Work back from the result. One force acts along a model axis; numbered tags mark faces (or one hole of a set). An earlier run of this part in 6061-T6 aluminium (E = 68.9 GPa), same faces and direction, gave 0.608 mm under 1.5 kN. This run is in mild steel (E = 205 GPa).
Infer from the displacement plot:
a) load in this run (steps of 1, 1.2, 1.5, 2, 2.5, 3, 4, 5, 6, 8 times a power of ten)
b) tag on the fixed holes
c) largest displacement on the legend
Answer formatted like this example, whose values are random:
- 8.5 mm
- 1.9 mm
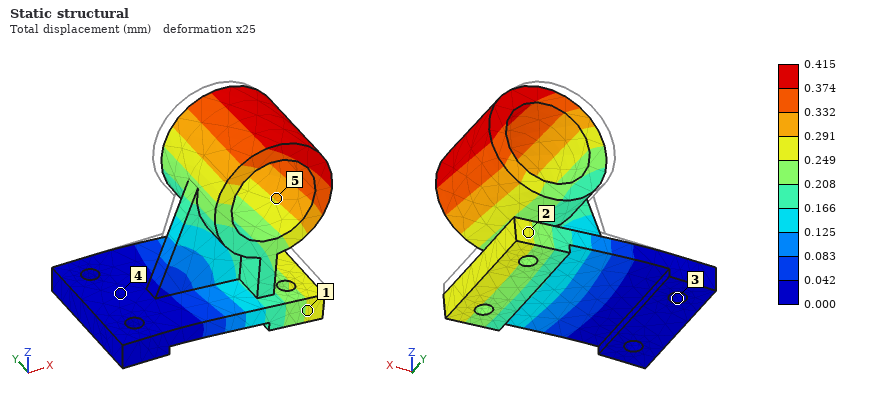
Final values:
- 3 kN
- 3
- 0.415 mm
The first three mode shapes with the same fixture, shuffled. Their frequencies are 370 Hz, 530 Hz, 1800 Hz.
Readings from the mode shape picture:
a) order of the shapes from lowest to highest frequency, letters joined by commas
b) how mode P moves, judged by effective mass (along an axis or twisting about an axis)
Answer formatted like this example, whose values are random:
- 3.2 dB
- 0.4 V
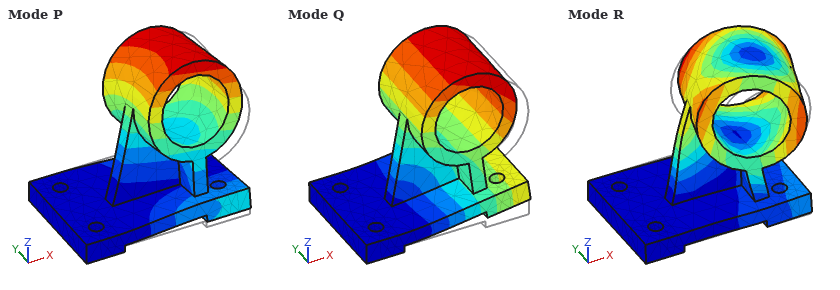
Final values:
- Q, P, R
- along Y
